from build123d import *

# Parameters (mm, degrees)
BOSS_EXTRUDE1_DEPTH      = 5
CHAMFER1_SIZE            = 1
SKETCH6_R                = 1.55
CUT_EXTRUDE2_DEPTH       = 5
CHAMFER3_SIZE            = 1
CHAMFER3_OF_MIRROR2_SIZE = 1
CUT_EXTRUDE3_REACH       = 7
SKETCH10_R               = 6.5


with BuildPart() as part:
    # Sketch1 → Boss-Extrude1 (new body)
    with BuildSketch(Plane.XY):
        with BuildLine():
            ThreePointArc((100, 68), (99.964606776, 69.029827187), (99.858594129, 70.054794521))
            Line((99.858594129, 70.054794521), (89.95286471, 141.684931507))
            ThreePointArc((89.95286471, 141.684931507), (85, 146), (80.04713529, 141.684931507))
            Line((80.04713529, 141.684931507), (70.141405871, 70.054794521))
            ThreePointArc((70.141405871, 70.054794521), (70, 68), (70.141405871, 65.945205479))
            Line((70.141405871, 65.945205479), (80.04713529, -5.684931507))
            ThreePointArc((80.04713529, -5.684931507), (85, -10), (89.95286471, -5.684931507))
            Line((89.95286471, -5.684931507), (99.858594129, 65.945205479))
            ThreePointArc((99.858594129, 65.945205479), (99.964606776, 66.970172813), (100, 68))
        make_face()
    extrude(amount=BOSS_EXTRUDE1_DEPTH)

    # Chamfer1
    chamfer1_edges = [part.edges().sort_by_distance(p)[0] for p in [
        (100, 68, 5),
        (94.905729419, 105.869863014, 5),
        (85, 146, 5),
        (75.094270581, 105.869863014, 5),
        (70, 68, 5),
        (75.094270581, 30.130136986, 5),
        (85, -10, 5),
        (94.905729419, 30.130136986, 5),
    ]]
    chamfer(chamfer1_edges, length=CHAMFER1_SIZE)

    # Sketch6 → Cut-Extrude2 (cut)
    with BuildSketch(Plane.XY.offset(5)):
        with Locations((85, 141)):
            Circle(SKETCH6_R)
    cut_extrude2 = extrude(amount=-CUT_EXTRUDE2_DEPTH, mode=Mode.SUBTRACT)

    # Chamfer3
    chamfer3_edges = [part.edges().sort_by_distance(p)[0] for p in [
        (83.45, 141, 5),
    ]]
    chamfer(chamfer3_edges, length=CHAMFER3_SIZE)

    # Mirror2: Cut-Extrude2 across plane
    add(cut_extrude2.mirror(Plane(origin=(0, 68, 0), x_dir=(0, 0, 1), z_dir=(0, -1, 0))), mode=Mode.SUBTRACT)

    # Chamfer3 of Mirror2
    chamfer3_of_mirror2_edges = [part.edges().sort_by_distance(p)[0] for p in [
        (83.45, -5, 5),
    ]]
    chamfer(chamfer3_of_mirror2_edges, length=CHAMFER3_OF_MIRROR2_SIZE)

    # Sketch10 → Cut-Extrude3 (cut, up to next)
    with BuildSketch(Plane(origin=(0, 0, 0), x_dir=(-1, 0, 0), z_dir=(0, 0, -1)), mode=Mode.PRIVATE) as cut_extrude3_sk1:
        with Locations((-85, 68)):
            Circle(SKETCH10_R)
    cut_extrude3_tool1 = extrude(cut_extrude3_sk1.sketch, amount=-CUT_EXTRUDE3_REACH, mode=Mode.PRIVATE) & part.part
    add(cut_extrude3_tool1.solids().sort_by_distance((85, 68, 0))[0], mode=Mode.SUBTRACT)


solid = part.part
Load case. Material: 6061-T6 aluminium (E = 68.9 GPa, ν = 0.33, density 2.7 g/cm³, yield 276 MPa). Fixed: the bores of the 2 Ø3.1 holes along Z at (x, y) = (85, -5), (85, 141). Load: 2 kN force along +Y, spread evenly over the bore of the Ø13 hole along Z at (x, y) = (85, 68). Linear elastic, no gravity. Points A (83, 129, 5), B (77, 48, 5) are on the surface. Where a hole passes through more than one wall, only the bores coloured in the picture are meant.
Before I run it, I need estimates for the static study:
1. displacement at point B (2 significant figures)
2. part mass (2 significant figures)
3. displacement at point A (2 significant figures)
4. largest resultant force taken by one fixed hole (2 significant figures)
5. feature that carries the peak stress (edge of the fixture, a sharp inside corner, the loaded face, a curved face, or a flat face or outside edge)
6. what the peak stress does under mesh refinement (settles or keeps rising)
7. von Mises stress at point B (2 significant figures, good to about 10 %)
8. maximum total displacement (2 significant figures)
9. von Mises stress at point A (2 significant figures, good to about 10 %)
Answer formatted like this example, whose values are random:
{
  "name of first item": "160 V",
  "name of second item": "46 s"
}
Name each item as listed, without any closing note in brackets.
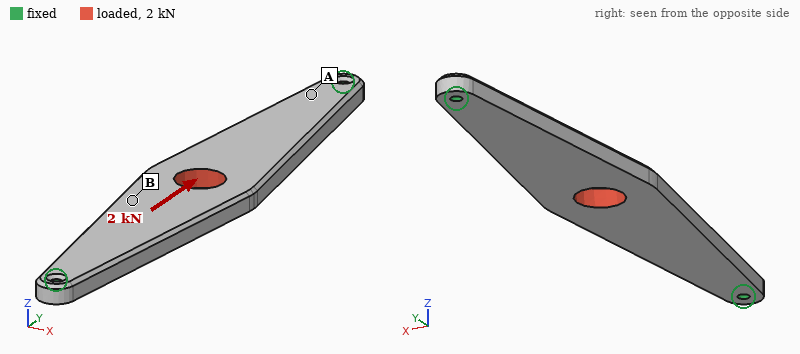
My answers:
{
  "displacement at point B": "10 µm",
  "part mass": "38 g",
  "displacement at point A": "3.8 µm",
  "largest resultant force taken by one fixed hole": "1.0 kN",
  "feature that carries the peak stress": "edge of the fixture",
  "what the peak stress does under mesh refinement": "keeps rising",
  "von Mises stress at point B": "8.0 MPa",
  "maximum total displacement": "13 µm",
  "von Mises stress at point A": "15 MPa"
}
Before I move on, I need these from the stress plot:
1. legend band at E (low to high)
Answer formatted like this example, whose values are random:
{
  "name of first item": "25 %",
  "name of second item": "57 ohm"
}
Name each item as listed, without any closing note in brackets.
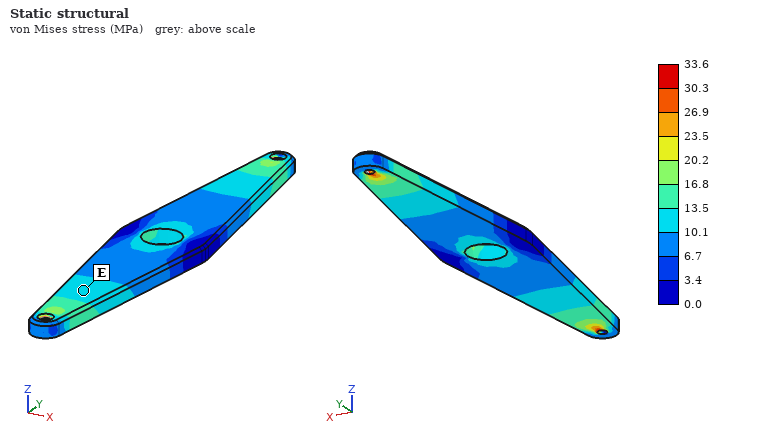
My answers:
{
  "legend band at E": "10.1 to 13.5 MPa"
}
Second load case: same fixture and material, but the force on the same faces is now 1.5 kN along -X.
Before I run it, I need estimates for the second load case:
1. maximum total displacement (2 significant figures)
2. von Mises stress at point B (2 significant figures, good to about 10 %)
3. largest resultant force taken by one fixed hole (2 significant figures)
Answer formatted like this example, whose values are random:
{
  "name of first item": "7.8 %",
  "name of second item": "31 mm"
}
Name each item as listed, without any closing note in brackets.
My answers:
{
  "maximum total displacement": "0.19 mm",
  "von Mises stress at point B": "40 MPa",
  "largest resultant force taken by one fixed hole": "750 N"
}
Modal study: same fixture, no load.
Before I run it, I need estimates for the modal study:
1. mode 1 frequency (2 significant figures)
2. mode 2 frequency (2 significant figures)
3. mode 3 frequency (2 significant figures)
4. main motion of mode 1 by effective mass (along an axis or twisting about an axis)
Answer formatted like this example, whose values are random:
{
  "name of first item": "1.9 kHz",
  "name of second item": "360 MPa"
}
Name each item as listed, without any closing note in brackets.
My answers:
{
  "mode 1 frequency": "960 Hz",
  "mode 2 frequency": "2900 Hz",
  "mode 3 frequency": "2900 Hz",
  "main motion of mode 1 by effective mass": "along Z"
}
